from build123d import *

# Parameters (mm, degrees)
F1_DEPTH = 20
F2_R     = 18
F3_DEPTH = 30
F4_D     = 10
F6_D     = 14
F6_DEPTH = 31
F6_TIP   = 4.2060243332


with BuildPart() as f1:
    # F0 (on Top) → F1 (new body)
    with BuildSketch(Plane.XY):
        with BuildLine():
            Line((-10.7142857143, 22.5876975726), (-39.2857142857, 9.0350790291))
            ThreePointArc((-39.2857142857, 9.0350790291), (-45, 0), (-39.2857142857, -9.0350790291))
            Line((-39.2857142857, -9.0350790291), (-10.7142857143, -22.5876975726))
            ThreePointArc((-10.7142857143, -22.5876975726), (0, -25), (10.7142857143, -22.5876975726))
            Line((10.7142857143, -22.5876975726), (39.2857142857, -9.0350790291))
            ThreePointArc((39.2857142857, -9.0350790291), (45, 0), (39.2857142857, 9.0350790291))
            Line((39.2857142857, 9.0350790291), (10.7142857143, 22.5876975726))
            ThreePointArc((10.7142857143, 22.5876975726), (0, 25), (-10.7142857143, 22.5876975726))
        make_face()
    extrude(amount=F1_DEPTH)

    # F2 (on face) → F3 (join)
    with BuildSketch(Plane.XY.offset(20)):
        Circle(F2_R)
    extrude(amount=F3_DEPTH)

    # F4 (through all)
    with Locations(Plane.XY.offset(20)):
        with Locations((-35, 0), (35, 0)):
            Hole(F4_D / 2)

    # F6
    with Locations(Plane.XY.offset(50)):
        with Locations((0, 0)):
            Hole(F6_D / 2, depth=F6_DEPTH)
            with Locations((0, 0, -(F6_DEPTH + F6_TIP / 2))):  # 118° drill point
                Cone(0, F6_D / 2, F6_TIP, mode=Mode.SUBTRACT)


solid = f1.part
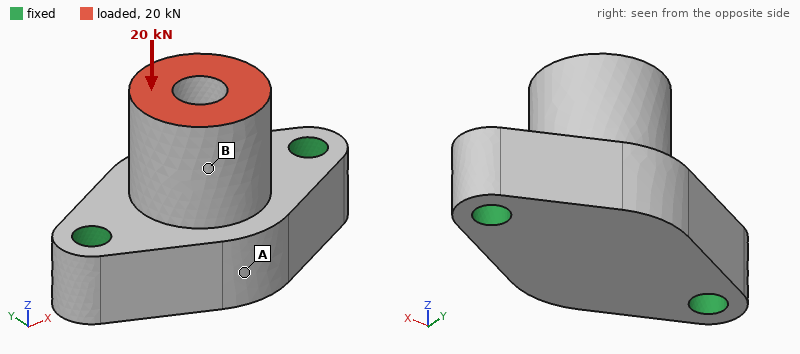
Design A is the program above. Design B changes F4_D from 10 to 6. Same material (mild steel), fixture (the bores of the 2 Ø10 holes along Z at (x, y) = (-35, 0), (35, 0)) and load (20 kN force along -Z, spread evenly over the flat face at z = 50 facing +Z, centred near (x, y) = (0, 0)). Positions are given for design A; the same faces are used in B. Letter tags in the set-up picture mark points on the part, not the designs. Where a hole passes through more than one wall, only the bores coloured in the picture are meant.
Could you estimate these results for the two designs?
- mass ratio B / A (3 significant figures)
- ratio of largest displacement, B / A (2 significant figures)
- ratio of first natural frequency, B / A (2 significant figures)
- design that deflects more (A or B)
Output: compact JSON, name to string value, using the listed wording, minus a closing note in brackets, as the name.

{"mass ratio B / A": "1.02", "ratio of largest displacement, B / A": "1.2", "ratio of first natural frequency, B / A": "0.90", "design that deflects more": "B"}
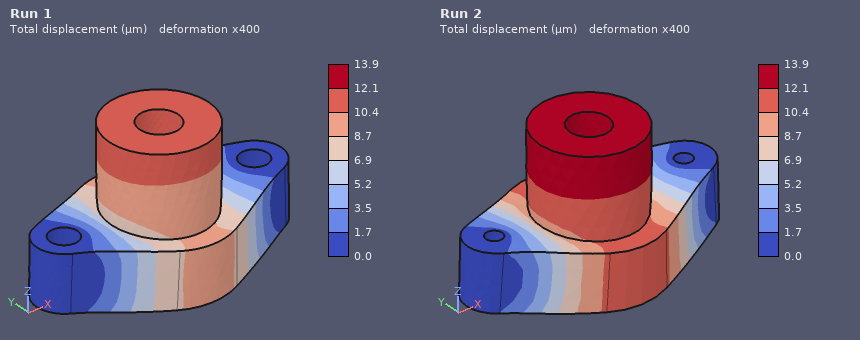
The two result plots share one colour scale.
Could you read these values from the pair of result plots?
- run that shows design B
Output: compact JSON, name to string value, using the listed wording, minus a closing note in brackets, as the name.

{"run that shows design B": "Run 2"}
